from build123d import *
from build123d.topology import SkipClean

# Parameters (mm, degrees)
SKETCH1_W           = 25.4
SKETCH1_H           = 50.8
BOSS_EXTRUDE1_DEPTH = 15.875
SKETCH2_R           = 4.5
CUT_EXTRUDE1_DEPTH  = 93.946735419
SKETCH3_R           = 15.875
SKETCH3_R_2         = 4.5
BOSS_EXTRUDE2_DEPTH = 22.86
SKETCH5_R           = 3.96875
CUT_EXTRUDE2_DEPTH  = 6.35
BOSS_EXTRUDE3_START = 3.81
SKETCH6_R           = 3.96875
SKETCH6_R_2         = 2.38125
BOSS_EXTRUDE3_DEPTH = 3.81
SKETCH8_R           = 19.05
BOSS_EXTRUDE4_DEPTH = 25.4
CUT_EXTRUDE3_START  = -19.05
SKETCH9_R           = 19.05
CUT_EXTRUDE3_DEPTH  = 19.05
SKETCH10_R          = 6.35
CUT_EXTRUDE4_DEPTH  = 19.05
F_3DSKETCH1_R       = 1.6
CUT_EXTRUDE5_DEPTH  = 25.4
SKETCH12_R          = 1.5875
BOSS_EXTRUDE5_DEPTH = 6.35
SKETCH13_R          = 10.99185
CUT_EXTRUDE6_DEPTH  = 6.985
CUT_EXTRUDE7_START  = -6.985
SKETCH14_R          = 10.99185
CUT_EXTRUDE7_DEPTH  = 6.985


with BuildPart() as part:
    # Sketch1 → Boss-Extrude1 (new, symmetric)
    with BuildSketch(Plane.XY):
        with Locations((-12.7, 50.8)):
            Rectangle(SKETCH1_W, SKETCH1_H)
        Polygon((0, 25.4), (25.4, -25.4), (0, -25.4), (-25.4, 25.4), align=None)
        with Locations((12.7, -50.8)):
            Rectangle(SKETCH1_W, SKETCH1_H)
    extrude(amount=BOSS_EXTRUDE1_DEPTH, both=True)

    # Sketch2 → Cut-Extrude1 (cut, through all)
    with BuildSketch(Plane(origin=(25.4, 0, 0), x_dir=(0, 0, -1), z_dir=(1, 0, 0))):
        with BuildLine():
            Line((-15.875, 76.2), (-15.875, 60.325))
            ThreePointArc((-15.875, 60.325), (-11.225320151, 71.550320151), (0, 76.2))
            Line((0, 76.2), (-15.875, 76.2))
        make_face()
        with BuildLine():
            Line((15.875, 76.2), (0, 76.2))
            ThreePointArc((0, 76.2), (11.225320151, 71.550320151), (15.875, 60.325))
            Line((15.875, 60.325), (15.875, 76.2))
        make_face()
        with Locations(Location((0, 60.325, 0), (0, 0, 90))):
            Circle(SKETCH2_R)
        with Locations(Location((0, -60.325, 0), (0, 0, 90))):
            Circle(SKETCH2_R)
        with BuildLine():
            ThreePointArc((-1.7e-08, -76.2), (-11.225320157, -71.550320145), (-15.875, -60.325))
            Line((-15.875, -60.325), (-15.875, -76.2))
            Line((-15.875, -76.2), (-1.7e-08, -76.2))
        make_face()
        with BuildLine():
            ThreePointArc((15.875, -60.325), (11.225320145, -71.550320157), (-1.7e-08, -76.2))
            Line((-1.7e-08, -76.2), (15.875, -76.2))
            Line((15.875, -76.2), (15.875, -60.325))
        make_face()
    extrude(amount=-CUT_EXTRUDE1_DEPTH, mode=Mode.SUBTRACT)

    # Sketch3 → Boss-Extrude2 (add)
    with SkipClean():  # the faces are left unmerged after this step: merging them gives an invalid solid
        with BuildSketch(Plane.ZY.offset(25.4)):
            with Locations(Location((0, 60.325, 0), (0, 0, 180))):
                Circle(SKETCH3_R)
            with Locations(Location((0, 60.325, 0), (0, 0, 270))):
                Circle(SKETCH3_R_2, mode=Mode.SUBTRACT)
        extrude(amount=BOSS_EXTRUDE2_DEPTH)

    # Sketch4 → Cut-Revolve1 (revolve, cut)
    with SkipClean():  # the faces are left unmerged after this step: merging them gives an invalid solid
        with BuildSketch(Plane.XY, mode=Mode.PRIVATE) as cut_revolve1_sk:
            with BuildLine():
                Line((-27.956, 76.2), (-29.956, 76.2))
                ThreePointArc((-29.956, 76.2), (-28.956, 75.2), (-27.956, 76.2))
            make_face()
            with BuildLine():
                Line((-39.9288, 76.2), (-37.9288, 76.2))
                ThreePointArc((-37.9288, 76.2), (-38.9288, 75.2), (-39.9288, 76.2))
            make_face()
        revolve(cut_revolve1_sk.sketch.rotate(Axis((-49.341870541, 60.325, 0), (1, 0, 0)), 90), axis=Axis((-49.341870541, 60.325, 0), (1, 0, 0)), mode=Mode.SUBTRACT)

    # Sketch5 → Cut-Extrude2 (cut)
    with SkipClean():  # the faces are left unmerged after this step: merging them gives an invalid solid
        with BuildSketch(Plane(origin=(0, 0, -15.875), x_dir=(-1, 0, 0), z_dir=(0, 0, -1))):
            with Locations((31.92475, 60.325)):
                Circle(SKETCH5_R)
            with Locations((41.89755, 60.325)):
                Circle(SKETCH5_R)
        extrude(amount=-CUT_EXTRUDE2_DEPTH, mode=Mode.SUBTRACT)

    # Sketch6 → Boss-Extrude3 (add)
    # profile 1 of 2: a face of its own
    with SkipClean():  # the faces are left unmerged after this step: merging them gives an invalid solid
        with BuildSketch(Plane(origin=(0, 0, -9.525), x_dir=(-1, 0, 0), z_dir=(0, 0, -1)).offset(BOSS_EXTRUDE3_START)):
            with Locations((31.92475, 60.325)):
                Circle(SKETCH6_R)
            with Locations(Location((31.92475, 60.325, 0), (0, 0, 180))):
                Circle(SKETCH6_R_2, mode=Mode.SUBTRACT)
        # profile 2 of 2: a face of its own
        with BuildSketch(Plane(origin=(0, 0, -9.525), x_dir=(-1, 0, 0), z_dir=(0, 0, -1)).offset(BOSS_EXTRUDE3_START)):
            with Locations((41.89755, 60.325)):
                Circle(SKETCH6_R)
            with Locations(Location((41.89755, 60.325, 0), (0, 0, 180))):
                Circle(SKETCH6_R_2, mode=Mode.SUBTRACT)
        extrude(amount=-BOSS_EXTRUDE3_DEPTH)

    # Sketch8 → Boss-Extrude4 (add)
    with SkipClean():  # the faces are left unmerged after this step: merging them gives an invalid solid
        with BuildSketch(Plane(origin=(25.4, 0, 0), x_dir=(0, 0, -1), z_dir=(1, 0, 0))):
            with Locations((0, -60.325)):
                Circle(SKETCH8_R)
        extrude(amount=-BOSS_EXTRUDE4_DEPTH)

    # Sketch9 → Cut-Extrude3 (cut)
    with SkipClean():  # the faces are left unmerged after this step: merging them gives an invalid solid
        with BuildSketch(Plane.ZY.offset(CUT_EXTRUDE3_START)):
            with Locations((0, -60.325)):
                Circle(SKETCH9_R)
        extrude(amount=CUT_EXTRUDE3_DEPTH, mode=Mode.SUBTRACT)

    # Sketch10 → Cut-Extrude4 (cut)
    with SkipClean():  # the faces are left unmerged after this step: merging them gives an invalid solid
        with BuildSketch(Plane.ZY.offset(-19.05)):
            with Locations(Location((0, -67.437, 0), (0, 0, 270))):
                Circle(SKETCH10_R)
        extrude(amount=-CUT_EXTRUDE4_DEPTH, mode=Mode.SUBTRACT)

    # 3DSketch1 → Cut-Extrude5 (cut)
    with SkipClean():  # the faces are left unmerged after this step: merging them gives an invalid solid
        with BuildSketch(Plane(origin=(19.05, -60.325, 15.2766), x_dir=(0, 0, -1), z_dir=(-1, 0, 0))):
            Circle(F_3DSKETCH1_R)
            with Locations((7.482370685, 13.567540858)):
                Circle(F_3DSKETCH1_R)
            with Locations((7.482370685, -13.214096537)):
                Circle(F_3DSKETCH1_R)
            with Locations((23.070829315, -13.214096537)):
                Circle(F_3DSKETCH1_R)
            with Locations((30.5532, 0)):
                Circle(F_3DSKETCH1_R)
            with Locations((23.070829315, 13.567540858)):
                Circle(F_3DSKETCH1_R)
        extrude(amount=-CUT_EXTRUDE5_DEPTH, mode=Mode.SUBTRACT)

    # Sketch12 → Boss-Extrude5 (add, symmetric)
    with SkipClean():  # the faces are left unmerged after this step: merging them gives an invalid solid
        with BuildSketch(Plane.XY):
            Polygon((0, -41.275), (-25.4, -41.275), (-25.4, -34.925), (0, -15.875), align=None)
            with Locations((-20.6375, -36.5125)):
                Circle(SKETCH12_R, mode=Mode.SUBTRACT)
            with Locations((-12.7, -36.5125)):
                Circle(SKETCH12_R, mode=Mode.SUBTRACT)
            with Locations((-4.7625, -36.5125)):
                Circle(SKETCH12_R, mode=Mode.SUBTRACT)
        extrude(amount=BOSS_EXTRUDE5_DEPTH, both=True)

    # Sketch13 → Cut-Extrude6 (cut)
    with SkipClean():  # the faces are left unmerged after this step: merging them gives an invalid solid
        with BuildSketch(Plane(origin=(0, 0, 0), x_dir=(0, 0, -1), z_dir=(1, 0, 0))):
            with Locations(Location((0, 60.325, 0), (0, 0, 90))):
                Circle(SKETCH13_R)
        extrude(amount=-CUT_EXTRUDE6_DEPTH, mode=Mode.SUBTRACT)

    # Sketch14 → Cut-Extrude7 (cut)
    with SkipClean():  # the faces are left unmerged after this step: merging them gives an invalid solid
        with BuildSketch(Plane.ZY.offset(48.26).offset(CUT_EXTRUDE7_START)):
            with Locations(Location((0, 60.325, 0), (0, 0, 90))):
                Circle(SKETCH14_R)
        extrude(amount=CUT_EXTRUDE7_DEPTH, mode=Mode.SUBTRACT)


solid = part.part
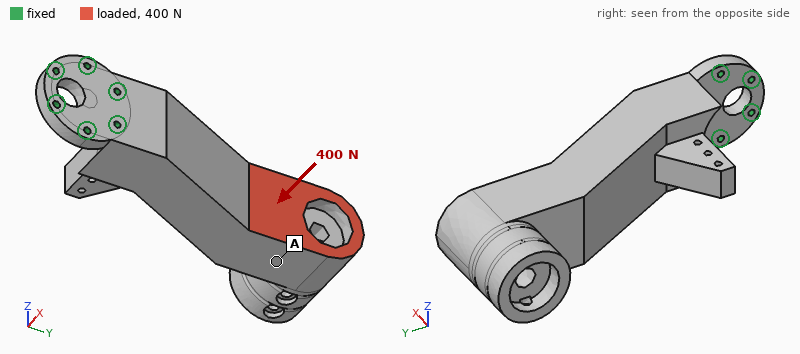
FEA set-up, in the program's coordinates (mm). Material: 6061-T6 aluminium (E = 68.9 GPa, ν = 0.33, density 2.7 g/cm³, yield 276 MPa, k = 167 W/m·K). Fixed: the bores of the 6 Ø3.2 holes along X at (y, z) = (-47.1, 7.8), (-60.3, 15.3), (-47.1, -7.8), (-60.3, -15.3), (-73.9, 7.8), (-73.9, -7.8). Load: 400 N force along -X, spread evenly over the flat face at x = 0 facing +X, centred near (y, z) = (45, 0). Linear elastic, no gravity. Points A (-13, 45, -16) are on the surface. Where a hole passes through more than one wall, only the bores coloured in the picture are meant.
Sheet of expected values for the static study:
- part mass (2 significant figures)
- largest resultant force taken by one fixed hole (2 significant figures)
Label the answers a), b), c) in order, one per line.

a) 310 g
b) 770 N
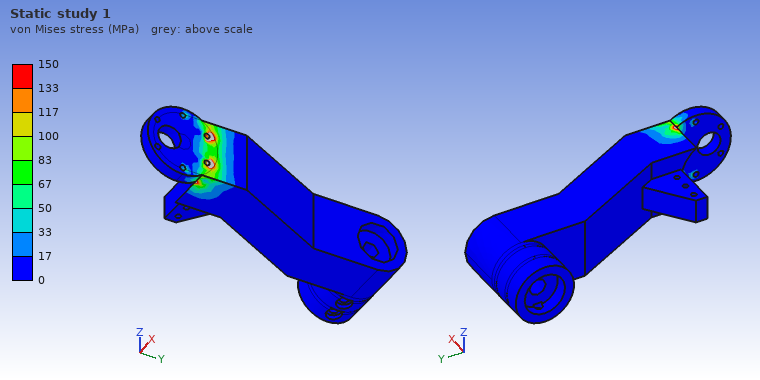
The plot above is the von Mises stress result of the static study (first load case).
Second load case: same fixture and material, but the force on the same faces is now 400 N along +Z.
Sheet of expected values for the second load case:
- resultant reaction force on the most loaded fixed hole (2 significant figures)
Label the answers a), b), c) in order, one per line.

a) 1.4 kN
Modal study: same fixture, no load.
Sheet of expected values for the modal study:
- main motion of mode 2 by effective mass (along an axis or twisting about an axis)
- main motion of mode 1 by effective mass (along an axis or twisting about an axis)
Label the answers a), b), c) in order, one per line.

a) along Z
b) along X
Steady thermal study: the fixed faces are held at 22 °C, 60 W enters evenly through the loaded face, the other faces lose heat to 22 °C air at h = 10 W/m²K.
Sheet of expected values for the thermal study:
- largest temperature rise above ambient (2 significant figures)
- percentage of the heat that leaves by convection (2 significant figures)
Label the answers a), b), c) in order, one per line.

a) 55 K
b) 13 %
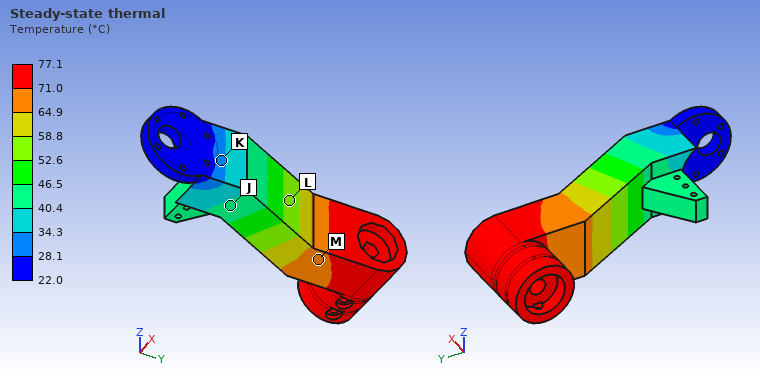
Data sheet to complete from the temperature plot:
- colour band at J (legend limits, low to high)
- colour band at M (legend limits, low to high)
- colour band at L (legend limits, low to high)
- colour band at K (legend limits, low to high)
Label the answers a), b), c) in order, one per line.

a) 40.4 to 46.5 °C
b) 64.9 to 71.0 °C
c) 52.6 to 58.8 °C
d) 28.1 to 34.3 °C
